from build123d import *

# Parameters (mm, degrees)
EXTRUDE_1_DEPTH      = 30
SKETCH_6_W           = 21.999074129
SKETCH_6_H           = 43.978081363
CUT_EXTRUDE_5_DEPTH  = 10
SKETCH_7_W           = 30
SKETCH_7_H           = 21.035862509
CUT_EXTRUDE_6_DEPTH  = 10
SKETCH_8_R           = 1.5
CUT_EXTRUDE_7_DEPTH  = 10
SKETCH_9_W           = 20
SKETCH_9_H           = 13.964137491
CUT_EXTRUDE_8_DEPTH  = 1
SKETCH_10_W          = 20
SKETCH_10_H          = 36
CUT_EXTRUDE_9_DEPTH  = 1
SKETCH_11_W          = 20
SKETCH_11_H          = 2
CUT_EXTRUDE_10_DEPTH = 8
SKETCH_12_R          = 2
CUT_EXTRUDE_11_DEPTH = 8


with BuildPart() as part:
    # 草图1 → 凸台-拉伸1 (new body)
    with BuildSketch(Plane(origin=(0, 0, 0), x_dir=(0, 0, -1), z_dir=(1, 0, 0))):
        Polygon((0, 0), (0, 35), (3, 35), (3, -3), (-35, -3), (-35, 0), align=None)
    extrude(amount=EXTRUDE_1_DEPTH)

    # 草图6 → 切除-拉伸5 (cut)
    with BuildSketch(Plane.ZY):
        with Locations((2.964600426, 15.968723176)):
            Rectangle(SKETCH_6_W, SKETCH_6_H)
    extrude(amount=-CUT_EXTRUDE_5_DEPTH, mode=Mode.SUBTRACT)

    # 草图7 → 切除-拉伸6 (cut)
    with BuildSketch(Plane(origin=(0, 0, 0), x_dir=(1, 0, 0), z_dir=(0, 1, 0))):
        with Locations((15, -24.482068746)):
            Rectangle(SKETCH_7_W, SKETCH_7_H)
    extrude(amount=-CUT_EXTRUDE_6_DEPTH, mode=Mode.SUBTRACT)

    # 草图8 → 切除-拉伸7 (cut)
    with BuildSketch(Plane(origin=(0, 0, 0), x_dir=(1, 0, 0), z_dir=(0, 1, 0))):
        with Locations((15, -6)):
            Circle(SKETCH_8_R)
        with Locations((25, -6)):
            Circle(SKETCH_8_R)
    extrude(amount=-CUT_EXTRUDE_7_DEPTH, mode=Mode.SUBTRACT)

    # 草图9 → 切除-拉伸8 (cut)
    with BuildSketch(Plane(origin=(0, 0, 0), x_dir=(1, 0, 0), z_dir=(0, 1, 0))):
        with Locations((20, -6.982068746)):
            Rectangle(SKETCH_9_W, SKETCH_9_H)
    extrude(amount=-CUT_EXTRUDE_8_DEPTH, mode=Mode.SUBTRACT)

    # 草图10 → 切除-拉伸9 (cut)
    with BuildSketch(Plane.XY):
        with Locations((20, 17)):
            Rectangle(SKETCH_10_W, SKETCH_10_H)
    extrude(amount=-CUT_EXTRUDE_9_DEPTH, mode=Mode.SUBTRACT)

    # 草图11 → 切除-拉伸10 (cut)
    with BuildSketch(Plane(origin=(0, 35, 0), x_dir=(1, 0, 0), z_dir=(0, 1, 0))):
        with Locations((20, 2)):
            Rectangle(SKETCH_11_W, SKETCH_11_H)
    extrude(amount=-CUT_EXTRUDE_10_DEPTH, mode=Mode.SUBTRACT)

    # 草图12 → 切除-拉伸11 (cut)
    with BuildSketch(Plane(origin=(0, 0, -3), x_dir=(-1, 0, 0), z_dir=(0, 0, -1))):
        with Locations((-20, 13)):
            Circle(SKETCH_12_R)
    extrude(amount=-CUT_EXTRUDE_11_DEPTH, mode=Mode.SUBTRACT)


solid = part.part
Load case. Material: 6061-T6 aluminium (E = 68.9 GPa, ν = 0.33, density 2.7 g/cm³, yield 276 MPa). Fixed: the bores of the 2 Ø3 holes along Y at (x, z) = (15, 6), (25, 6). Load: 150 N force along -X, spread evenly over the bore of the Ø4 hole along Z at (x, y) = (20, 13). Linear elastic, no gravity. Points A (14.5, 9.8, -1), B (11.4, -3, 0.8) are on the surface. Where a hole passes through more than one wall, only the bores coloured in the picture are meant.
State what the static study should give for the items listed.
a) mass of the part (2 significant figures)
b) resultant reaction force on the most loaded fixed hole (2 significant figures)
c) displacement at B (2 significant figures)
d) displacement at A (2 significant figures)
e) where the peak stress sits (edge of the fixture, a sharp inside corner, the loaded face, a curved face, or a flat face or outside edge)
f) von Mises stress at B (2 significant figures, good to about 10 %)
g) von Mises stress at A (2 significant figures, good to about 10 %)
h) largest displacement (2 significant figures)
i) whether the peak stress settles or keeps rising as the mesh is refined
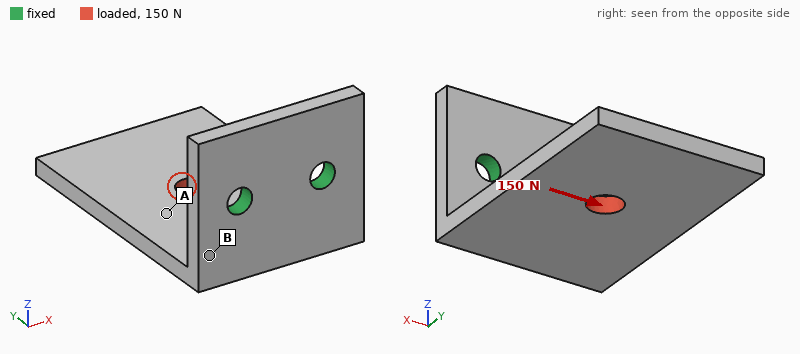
4.7 g
210 N
0.022 mm
0.059 mm
edge of the fixture
34 MPa
13 MPa
0.14 mm
keeps rising
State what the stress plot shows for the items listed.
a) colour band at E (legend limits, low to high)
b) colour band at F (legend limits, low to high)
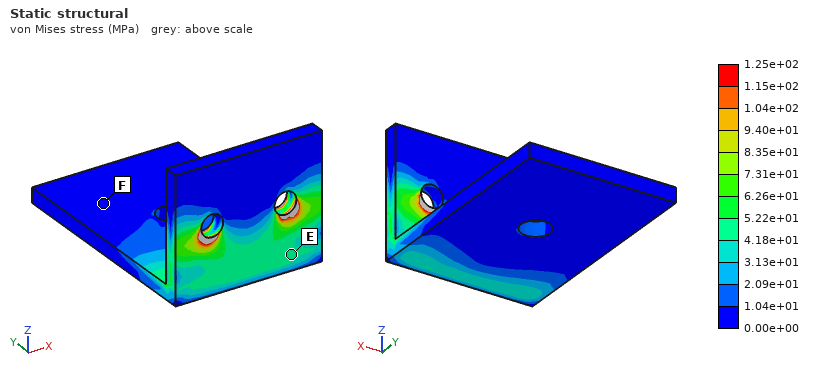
4.18e+01 to 5.22e+01 MPa
0.00e+00 to 1.04e+01 MPa
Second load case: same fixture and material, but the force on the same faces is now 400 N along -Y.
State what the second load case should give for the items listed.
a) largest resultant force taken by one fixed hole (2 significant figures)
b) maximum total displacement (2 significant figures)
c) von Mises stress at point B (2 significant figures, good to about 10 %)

200 N
0.33 mm
77 MPa
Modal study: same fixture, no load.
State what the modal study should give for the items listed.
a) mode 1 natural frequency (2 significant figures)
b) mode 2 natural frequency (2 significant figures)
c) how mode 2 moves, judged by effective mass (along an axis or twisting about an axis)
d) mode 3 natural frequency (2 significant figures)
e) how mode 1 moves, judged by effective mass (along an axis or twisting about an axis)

1400 Hz
3600 Hz
along X
6000 Hz
along Z
